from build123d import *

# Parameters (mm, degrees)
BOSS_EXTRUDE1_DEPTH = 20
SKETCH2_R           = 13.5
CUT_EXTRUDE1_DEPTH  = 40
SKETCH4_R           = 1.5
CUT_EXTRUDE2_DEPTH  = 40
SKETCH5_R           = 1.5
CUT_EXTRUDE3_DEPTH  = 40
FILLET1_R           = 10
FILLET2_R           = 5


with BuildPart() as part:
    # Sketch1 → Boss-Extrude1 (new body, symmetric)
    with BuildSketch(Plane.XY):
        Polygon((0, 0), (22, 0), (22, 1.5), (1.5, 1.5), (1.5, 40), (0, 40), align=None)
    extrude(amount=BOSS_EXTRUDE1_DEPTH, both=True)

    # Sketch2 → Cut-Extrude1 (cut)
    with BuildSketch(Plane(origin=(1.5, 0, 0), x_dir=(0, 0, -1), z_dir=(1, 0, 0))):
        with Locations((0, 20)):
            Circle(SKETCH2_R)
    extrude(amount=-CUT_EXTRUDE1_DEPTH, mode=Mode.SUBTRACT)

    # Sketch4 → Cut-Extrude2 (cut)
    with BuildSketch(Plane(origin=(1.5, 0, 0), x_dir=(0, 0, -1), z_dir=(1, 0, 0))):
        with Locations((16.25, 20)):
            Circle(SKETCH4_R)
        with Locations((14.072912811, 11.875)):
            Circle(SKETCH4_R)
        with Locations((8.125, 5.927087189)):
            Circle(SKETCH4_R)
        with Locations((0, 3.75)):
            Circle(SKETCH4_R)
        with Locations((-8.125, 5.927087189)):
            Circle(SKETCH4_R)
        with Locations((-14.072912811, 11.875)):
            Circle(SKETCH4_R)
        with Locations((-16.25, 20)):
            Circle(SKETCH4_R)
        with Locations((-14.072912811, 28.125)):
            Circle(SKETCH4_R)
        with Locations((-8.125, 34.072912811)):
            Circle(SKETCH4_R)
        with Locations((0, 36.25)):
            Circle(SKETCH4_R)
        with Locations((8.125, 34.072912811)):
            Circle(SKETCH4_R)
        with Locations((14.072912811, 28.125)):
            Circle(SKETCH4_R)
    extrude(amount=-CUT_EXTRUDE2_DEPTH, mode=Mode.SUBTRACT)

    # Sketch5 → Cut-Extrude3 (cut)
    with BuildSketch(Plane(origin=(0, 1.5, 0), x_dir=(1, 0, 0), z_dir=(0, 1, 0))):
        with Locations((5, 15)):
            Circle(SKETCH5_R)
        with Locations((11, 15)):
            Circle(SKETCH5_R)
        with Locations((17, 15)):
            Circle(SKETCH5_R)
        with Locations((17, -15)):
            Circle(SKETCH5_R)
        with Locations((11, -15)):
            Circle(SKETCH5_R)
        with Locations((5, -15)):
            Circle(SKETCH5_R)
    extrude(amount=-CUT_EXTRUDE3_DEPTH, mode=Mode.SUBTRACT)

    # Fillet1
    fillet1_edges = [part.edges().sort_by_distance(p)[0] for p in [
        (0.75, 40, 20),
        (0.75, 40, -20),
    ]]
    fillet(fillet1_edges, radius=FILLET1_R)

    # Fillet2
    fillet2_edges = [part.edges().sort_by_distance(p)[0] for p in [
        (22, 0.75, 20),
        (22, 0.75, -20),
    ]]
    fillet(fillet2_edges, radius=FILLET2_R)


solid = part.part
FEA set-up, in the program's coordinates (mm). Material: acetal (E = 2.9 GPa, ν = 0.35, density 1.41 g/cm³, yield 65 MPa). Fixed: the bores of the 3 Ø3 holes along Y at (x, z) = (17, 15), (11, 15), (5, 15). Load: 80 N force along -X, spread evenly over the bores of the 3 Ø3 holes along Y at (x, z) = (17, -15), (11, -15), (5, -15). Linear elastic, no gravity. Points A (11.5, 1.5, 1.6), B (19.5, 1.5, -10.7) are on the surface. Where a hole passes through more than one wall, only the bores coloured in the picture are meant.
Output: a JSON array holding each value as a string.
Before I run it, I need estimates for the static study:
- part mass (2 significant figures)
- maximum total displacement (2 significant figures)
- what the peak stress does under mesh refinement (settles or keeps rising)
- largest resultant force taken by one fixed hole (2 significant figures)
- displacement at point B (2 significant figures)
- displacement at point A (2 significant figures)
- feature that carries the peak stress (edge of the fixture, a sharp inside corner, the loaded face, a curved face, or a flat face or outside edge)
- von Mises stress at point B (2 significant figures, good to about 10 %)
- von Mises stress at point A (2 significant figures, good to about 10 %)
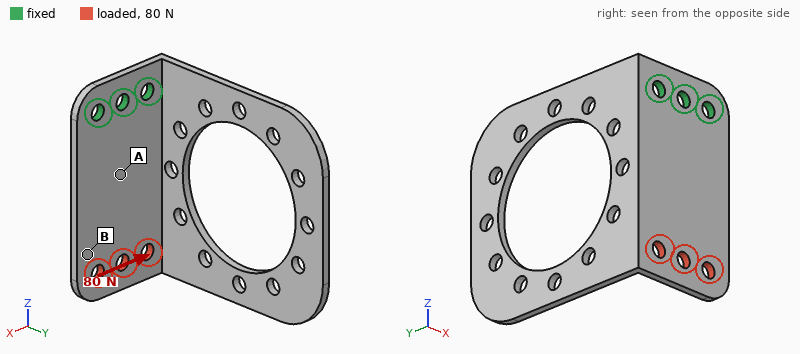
["3.5 g", "0.38 mm", "keeps rising", "170 N", "0.26 mm", "0.095 mm", "edge of the fixture", "2.9 MPa", "6.7 MPa"]
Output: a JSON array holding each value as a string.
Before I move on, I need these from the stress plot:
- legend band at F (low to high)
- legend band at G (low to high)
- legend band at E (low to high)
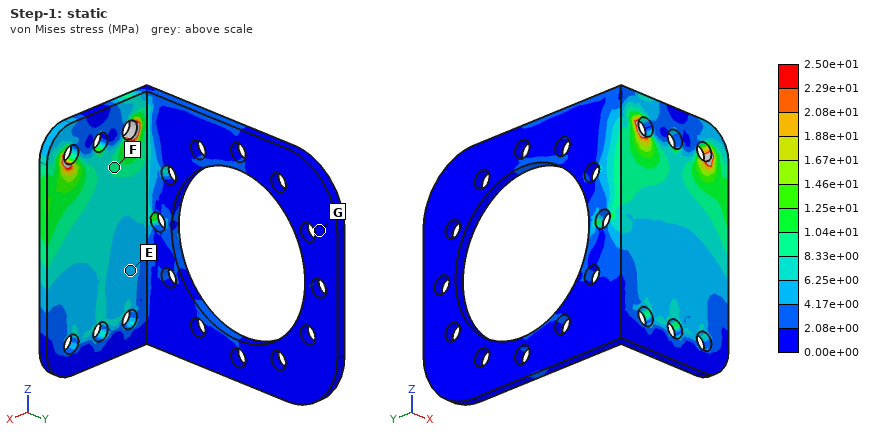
["8.33e+00 to 1.04e+01 MPa", "0.00e+00 to 2.08e+00 MPa", "4.17e+00 to 6.25e+00 MPa"]
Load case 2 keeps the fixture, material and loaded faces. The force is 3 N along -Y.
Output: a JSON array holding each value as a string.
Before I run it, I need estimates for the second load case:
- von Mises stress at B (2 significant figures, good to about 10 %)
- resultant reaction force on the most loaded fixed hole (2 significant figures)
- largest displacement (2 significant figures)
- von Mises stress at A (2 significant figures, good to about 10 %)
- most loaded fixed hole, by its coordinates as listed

["1.1 MPa", "1.9 N", "0.59 mm", "1.4 MPa", "(11, 15)"]
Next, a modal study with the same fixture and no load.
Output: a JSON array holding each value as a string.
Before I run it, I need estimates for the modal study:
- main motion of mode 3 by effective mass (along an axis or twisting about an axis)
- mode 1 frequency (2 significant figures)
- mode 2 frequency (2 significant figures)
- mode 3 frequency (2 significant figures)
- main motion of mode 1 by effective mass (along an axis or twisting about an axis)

["twisting about Y", "160 Hz", "290 Hz", "410 Hz", "along X"]
